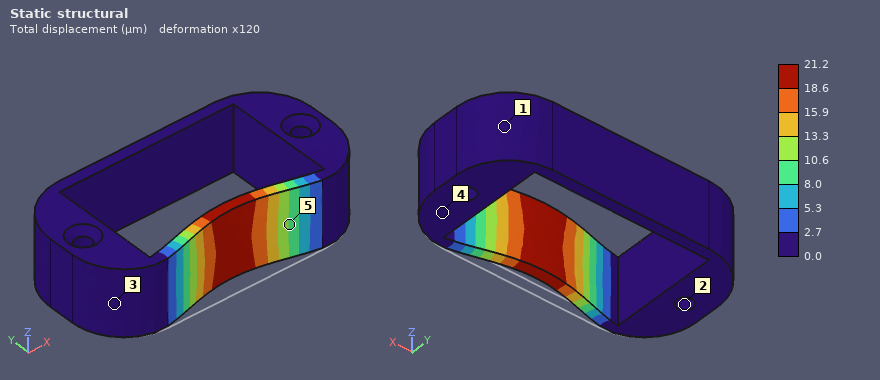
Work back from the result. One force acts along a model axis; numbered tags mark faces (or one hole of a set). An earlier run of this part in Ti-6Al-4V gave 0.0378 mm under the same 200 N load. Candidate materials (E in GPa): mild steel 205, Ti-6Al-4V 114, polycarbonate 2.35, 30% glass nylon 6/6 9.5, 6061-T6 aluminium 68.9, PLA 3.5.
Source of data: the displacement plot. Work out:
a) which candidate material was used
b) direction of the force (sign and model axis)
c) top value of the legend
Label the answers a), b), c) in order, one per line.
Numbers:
a) mild steel
b) +Y
c) 21.2 µm
